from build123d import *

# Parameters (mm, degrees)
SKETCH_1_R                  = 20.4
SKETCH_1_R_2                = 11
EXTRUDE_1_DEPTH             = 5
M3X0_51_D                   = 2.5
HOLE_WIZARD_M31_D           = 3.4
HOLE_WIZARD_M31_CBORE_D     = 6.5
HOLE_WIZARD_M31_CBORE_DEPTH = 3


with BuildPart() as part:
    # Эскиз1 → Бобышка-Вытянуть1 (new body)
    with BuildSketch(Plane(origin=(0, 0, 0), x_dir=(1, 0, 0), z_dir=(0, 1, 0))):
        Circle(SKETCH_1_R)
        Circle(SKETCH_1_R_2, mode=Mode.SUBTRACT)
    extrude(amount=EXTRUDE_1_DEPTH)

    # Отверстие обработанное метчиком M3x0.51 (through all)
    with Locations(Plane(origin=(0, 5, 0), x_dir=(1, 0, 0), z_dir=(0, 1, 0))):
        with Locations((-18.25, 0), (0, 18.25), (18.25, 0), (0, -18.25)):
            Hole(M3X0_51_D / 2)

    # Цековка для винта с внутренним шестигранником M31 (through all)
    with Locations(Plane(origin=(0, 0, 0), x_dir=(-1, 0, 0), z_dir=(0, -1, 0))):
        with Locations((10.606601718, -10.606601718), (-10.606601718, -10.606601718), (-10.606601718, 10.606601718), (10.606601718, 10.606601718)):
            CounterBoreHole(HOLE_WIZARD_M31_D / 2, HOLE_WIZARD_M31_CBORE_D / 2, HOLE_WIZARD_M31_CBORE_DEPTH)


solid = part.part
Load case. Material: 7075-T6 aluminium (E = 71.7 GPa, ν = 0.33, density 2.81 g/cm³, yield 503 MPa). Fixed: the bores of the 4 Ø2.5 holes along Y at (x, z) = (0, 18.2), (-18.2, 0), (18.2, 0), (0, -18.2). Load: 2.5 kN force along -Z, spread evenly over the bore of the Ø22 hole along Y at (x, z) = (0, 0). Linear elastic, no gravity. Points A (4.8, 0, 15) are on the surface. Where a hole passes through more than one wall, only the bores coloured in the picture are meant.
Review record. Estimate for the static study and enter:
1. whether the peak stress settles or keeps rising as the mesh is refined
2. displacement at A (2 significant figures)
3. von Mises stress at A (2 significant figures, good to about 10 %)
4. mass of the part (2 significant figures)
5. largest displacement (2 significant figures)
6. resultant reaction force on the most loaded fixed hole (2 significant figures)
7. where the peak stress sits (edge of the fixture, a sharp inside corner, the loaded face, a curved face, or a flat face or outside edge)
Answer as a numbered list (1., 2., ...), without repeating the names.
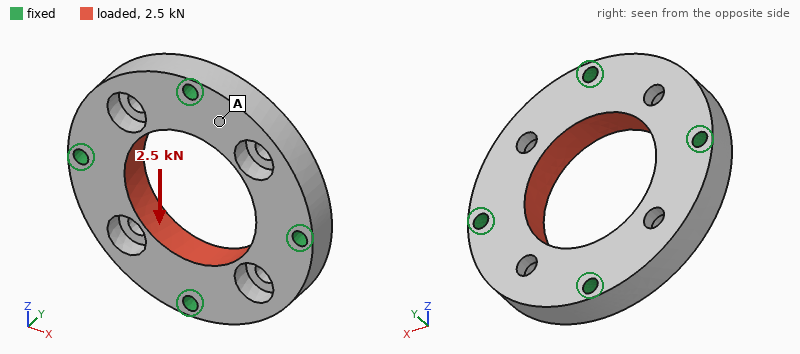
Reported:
1. keeps rising
2. 1.6 µm
3. 11 MPa
4. 11 g
5. 6.1 µm
6. 630 N
7. edge of the fixture
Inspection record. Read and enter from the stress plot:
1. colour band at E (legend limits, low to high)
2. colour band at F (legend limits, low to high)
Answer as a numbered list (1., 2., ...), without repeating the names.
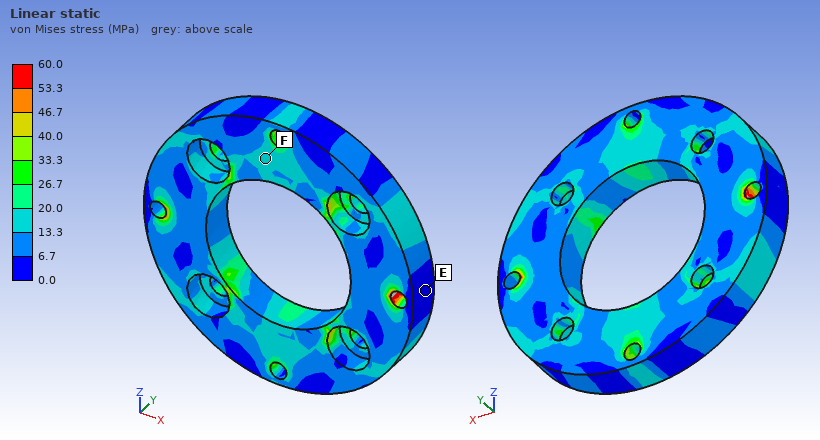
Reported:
1. 0.0 to 6.7 MPa
2. 13.3 to 20.0 MPa
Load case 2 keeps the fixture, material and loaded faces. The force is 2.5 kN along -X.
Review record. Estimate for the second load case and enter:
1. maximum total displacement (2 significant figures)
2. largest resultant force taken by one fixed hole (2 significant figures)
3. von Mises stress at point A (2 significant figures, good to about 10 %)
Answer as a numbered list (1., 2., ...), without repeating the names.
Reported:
1. 6.0 µm
2. 630 N
3. 5.3 MPa
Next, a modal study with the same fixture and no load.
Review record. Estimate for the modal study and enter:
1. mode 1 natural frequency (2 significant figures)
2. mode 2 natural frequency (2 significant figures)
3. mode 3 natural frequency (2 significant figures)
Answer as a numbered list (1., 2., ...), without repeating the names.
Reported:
1. 27 kHz
2. 29 kHz
3. 29 kHz
